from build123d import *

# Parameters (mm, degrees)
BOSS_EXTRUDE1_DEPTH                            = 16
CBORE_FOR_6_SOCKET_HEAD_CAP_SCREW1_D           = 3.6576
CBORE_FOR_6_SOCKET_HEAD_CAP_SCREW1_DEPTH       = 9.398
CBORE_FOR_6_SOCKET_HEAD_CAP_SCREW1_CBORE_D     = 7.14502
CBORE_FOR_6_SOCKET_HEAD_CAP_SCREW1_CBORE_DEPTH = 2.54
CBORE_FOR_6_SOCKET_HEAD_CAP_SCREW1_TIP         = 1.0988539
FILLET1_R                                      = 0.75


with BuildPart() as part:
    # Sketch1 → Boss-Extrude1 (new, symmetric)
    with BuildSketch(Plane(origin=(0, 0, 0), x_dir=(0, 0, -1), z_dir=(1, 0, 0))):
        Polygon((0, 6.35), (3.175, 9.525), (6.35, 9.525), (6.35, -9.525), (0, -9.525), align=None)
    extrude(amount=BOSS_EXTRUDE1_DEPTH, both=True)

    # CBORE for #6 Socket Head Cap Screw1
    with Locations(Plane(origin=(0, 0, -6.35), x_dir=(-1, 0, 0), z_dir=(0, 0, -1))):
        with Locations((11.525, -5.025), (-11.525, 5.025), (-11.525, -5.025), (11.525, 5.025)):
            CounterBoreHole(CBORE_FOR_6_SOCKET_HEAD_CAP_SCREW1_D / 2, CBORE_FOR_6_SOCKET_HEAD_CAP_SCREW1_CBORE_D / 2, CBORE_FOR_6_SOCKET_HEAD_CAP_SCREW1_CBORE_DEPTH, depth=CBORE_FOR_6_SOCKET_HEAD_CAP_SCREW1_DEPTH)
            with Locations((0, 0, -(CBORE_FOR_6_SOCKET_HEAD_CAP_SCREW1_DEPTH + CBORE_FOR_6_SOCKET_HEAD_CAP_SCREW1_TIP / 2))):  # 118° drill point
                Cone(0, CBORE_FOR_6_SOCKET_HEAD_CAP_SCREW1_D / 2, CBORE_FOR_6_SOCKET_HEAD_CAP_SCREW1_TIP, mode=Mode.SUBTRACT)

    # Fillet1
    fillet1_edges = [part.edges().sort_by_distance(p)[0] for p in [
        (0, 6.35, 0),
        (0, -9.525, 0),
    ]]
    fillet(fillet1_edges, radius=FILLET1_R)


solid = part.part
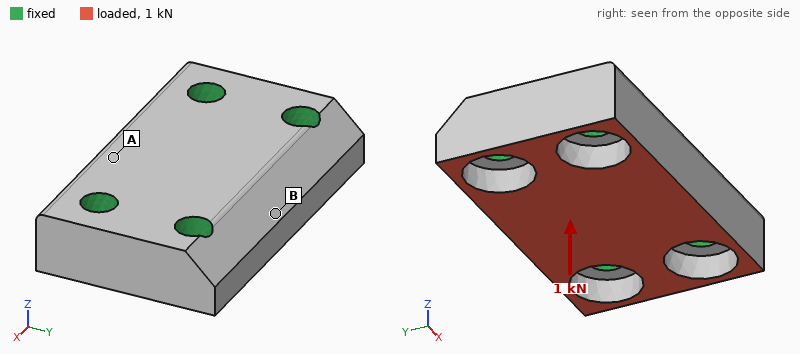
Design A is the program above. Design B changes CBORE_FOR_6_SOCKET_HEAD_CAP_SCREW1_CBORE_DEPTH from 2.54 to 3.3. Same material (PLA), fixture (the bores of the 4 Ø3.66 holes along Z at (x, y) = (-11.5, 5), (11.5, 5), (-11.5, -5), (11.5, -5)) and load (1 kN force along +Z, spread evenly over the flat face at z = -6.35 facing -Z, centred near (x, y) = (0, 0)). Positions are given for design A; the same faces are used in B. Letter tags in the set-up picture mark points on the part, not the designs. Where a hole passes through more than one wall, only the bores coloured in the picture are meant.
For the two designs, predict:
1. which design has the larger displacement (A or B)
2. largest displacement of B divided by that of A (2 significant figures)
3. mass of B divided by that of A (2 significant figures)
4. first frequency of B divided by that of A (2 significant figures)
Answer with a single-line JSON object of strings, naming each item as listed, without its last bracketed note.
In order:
{"which design has the larger displacement": "B", "largest displacement of B divided by that of A": "1.1", "mass of B divided by that of A": "0.97", "first frequency of B divided by that of A": "0.93"}
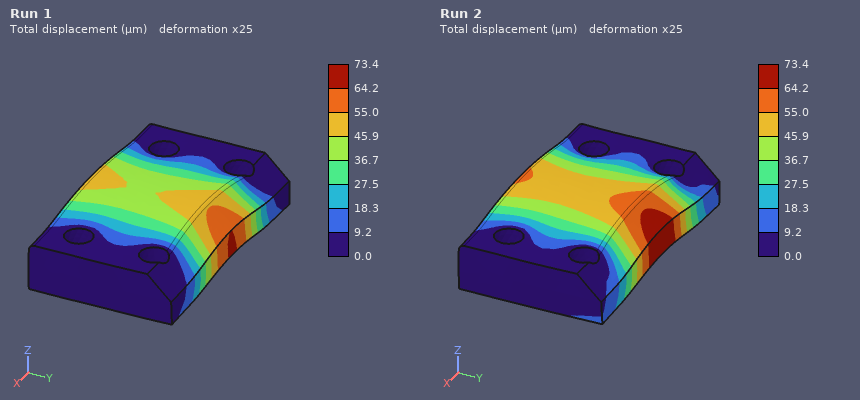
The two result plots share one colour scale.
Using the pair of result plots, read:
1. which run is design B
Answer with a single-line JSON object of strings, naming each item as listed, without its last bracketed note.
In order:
{"which run is design B": "Run 2"}
